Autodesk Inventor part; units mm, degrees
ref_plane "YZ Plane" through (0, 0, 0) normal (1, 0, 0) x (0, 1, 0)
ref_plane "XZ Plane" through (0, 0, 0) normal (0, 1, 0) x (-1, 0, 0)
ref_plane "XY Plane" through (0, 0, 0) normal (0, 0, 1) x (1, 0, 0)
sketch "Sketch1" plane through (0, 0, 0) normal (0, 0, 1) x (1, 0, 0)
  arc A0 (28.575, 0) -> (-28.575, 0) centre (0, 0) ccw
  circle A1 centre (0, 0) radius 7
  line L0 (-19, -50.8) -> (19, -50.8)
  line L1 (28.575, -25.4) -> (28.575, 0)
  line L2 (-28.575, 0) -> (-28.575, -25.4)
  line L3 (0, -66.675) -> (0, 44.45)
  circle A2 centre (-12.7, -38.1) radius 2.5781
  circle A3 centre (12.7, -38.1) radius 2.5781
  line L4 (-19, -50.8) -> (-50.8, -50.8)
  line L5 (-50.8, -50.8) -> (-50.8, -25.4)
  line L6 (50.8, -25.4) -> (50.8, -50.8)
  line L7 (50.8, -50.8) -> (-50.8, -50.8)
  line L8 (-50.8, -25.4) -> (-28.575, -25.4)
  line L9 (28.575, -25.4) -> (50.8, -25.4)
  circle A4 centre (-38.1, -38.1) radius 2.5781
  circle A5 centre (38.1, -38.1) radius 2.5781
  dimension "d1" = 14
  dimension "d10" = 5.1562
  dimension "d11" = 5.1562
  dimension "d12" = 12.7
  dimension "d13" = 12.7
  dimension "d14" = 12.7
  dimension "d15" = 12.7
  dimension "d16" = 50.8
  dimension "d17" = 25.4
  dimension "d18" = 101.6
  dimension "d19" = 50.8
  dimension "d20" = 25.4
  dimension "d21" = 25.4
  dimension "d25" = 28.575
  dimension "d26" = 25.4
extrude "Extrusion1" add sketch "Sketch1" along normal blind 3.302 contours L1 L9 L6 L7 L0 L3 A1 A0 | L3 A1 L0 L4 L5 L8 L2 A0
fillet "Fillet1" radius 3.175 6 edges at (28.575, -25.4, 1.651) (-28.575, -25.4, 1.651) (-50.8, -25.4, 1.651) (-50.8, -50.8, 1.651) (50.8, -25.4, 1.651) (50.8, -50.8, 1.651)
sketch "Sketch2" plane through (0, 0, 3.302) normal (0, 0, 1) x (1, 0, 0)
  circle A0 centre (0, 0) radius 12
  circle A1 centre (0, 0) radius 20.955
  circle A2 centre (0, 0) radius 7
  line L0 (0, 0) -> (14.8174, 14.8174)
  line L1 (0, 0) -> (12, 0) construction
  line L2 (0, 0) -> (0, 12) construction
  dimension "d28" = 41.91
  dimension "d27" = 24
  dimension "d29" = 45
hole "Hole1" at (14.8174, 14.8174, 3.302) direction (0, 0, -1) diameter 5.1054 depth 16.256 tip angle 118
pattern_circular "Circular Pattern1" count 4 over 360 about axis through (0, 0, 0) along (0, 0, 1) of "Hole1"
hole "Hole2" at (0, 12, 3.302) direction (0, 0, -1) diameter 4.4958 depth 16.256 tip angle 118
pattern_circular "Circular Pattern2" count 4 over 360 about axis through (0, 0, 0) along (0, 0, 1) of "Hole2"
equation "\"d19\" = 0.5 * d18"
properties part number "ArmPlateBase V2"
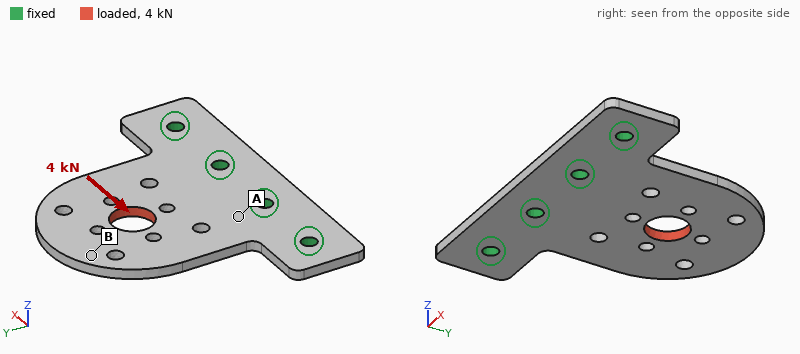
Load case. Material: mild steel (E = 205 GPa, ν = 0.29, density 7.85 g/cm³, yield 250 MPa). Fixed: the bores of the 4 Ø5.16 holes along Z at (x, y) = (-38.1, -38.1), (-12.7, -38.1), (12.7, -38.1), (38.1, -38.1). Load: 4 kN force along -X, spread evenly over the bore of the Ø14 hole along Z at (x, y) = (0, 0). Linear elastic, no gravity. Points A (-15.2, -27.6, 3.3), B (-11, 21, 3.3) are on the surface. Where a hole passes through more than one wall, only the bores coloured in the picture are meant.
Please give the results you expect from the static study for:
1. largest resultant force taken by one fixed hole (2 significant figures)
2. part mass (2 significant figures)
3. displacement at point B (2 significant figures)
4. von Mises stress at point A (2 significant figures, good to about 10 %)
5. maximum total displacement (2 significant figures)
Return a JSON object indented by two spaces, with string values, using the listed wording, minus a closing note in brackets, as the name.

{
  "largest resultant force taken by one fixed hole": "1.8 kN",
  "part mass": "130 g",
  "displacement at point B": "26 µm",
  "von Mises stress at point A": "25 MPa",
  "maximum total displacement": "27 µm"
}
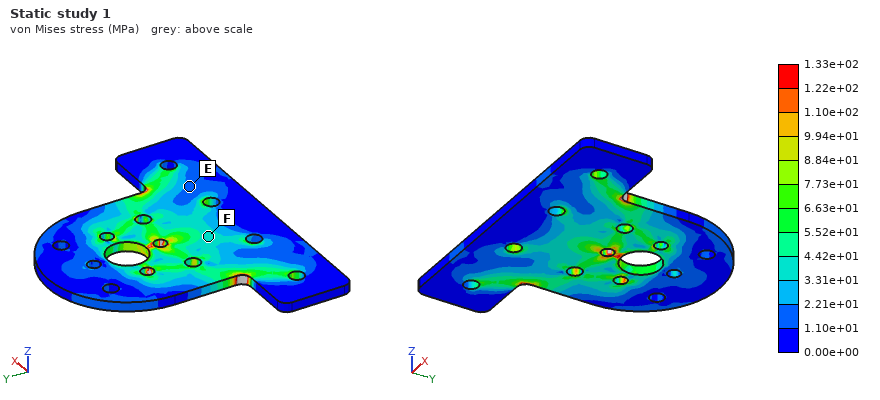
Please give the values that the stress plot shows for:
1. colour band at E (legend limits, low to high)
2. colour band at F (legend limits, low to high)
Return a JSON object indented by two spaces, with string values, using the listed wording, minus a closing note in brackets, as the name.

{
  "colour band at E": "1.10e+01 to 2.21e+01 MPa",
  "colour band at F": "3.31e+01 to 4.42e+01 MPa"
}
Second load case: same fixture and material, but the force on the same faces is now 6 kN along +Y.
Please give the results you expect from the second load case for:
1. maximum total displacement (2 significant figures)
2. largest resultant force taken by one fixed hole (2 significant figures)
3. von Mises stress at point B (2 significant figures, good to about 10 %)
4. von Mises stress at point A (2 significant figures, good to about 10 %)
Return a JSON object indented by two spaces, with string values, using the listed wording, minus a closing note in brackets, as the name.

{
  "maximum total displacement": "13 µm",
  "largest resultant force taken by one fixed hole": "2.3 kN",
  "von Mises stress at point B": "16 MPa",
  "von Mises stress at point A": "30 MPa"
}
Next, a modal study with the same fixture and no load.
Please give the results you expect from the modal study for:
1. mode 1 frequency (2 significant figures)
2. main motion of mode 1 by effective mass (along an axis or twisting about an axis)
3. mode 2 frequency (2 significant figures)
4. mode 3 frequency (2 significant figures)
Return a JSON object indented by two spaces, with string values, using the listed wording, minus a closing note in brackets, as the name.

{
  "mode 1 frequency": "790 Hz",
  "main motion of mode 1 by effective mass": "along Z",
  "mode 2 frequency": "2200 Hz",
  "mode 3 frequency": "4100 Hz"
}
